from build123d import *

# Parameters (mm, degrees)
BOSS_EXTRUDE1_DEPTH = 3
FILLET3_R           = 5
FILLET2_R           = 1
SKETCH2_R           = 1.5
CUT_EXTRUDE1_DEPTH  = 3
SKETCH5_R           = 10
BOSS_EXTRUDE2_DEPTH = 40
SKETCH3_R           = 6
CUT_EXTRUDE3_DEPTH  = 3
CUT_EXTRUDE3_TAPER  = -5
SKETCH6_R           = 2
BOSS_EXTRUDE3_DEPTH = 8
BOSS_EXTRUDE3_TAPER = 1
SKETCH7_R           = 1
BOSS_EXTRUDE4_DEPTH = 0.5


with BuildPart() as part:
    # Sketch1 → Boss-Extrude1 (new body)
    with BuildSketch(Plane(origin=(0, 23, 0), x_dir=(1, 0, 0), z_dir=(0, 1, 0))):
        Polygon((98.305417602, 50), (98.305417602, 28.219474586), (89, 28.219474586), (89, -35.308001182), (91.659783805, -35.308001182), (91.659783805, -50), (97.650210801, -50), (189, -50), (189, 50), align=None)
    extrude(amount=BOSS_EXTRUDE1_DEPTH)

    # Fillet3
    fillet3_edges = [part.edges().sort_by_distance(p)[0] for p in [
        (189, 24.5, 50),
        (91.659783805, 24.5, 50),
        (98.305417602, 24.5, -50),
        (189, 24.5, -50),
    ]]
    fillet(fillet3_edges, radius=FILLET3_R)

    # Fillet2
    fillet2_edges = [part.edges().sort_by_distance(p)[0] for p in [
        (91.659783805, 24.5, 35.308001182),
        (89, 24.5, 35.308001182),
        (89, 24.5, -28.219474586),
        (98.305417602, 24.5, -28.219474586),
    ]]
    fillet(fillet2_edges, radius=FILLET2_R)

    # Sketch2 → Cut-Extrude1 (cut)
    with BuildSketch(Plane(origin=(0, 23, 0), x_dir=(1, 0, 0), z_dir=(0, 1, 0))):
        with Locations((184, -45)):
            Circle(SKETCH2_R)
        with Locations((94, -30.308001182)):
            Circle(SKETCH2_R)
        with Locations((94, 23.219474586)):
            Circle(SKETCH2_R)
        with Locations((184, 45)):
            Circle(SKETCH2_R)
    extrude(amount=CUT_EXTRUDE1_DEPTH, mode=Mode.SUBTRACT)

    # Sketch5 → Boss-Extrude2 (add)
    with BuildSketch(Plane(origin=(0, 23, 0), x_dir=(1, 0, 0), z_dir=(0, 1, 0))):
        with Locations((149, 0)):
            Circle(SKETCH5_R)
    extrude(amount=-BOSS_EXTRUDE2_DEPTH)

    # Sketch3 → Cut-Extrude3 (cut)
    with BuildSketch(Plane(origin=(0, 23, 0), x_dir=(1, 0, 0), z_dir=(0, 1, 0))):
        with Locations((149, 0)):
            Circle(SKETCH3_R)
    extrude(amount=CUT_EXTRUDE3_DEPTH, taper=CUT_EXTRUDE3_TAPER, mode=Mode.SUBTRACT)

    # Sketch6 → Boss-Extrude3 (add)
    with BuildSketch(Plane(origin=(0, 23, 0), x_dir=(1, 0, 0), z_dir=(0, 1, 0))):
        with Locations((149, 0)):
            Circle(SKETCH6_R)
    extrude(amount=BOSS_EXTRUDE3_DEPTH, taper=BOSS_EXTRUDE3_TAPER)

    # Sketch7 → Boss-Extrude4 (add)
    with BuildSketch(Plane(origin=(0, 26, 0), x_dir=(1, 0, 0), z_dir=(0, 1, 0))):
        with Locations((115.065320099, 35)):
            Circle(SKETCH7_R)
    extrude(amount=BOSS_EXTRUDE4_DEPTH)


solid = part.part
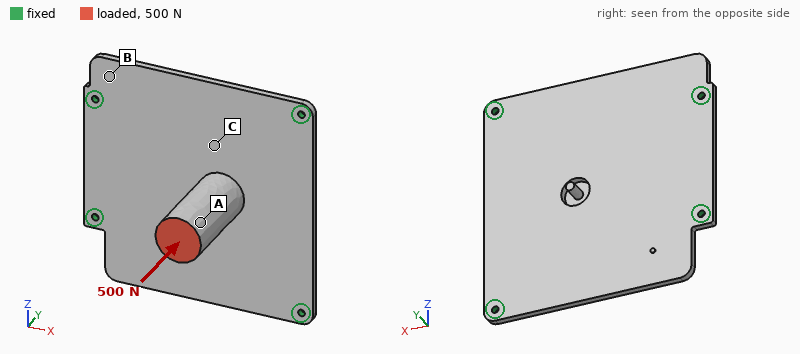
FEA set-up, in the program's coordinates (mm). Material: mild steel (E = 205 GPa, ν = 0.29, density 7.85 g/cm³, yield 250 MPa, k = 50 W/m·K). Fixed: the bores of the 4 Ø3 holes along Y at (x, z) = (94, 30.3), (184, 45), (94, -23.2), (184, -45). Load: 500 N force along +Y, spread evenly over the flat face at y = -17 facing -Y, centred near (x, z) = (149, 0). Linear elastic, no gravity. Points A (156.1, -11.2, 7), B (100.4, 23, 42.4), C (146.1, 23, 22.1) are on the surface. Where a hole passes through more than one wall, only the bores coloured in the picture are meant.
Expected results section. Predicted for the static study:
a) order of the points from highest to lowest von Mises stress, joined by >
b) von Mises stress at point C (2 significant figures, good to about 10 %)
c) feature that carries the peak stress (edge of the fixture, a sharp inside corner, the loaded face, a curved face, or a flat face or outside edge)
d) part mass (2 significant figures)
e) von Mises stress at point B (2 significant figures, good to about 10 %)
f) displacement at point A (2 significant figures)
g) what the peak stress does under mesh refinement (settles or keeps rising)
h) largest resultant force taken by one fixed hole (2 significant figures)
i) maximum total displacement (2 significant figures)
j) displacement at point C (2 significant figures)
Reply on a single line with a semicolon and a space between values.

C > B > A; 30 MPa; edge of the fixture; 330 g; 16 MPa; 88 µm; keeps rising; 150 N; 88 µm; 72 µm
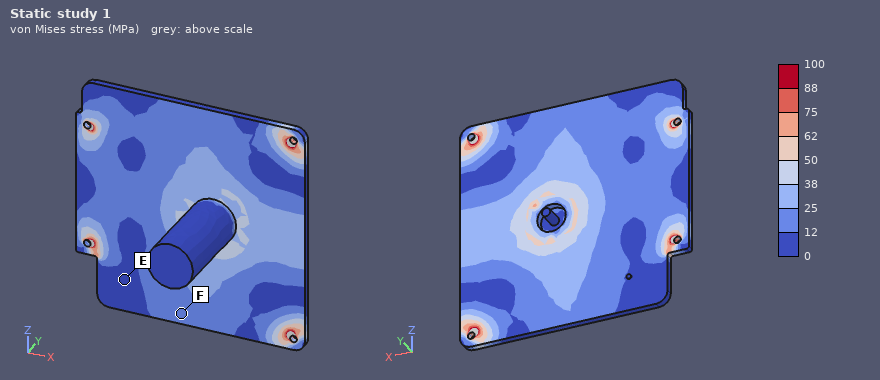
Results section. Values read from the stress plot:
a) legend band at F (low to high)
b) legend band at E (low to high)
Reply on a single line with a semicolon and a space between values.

12 to 25 MPa; 0 to 12 MPa
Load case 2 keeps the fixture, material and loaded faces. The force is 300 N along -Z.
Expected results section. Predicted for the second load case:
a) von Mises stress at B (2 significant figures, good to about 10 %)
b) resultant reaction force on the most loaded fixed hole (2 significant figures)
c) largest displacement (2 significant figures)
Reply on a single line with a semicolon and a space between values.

9.6 MPa; 150 N; 0.12 mm
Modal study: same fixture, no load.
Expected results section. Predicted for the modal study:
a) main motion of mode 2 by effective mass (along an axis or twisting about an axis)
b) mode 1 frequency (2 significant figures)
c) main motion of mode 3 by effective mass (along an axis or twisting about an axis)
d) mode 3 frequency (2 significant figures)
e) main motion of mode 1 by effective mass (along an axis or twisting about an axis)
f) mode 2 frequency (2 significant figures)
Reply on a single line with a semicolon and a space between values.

along Z; 920 Hz; along X; 1300 Hz; along Y; 1200 Hz
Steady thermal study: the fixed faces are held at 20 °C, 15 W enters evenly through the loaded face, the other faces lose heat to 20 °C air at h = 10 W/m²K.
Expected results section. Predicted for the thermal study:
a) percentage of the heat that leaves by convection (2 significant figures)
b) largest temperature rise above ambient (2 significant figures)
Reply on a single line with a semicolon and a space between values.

32 %; 75 K
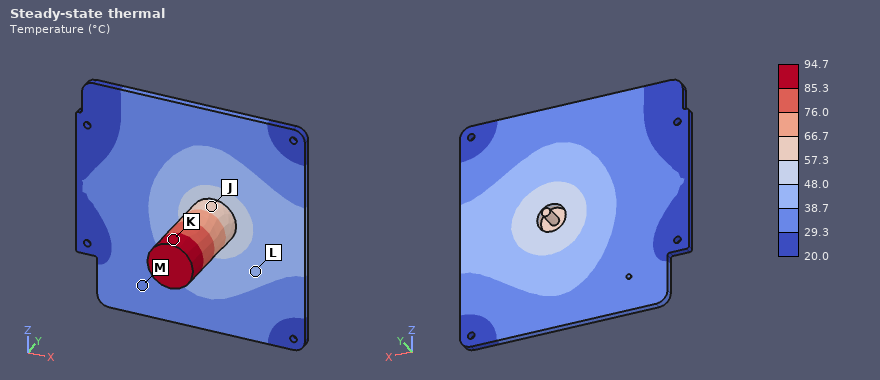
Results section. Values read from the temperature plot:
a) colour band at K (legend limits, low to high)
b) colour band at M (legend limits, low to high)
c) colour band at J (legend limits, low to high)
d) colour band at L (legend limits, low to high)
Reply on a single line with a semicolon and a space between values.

85.3 to 94.7 °C; 29.3 to 38.7 °C; 57.3 to 66.7 °C; 38.7 to 48.0 °C
